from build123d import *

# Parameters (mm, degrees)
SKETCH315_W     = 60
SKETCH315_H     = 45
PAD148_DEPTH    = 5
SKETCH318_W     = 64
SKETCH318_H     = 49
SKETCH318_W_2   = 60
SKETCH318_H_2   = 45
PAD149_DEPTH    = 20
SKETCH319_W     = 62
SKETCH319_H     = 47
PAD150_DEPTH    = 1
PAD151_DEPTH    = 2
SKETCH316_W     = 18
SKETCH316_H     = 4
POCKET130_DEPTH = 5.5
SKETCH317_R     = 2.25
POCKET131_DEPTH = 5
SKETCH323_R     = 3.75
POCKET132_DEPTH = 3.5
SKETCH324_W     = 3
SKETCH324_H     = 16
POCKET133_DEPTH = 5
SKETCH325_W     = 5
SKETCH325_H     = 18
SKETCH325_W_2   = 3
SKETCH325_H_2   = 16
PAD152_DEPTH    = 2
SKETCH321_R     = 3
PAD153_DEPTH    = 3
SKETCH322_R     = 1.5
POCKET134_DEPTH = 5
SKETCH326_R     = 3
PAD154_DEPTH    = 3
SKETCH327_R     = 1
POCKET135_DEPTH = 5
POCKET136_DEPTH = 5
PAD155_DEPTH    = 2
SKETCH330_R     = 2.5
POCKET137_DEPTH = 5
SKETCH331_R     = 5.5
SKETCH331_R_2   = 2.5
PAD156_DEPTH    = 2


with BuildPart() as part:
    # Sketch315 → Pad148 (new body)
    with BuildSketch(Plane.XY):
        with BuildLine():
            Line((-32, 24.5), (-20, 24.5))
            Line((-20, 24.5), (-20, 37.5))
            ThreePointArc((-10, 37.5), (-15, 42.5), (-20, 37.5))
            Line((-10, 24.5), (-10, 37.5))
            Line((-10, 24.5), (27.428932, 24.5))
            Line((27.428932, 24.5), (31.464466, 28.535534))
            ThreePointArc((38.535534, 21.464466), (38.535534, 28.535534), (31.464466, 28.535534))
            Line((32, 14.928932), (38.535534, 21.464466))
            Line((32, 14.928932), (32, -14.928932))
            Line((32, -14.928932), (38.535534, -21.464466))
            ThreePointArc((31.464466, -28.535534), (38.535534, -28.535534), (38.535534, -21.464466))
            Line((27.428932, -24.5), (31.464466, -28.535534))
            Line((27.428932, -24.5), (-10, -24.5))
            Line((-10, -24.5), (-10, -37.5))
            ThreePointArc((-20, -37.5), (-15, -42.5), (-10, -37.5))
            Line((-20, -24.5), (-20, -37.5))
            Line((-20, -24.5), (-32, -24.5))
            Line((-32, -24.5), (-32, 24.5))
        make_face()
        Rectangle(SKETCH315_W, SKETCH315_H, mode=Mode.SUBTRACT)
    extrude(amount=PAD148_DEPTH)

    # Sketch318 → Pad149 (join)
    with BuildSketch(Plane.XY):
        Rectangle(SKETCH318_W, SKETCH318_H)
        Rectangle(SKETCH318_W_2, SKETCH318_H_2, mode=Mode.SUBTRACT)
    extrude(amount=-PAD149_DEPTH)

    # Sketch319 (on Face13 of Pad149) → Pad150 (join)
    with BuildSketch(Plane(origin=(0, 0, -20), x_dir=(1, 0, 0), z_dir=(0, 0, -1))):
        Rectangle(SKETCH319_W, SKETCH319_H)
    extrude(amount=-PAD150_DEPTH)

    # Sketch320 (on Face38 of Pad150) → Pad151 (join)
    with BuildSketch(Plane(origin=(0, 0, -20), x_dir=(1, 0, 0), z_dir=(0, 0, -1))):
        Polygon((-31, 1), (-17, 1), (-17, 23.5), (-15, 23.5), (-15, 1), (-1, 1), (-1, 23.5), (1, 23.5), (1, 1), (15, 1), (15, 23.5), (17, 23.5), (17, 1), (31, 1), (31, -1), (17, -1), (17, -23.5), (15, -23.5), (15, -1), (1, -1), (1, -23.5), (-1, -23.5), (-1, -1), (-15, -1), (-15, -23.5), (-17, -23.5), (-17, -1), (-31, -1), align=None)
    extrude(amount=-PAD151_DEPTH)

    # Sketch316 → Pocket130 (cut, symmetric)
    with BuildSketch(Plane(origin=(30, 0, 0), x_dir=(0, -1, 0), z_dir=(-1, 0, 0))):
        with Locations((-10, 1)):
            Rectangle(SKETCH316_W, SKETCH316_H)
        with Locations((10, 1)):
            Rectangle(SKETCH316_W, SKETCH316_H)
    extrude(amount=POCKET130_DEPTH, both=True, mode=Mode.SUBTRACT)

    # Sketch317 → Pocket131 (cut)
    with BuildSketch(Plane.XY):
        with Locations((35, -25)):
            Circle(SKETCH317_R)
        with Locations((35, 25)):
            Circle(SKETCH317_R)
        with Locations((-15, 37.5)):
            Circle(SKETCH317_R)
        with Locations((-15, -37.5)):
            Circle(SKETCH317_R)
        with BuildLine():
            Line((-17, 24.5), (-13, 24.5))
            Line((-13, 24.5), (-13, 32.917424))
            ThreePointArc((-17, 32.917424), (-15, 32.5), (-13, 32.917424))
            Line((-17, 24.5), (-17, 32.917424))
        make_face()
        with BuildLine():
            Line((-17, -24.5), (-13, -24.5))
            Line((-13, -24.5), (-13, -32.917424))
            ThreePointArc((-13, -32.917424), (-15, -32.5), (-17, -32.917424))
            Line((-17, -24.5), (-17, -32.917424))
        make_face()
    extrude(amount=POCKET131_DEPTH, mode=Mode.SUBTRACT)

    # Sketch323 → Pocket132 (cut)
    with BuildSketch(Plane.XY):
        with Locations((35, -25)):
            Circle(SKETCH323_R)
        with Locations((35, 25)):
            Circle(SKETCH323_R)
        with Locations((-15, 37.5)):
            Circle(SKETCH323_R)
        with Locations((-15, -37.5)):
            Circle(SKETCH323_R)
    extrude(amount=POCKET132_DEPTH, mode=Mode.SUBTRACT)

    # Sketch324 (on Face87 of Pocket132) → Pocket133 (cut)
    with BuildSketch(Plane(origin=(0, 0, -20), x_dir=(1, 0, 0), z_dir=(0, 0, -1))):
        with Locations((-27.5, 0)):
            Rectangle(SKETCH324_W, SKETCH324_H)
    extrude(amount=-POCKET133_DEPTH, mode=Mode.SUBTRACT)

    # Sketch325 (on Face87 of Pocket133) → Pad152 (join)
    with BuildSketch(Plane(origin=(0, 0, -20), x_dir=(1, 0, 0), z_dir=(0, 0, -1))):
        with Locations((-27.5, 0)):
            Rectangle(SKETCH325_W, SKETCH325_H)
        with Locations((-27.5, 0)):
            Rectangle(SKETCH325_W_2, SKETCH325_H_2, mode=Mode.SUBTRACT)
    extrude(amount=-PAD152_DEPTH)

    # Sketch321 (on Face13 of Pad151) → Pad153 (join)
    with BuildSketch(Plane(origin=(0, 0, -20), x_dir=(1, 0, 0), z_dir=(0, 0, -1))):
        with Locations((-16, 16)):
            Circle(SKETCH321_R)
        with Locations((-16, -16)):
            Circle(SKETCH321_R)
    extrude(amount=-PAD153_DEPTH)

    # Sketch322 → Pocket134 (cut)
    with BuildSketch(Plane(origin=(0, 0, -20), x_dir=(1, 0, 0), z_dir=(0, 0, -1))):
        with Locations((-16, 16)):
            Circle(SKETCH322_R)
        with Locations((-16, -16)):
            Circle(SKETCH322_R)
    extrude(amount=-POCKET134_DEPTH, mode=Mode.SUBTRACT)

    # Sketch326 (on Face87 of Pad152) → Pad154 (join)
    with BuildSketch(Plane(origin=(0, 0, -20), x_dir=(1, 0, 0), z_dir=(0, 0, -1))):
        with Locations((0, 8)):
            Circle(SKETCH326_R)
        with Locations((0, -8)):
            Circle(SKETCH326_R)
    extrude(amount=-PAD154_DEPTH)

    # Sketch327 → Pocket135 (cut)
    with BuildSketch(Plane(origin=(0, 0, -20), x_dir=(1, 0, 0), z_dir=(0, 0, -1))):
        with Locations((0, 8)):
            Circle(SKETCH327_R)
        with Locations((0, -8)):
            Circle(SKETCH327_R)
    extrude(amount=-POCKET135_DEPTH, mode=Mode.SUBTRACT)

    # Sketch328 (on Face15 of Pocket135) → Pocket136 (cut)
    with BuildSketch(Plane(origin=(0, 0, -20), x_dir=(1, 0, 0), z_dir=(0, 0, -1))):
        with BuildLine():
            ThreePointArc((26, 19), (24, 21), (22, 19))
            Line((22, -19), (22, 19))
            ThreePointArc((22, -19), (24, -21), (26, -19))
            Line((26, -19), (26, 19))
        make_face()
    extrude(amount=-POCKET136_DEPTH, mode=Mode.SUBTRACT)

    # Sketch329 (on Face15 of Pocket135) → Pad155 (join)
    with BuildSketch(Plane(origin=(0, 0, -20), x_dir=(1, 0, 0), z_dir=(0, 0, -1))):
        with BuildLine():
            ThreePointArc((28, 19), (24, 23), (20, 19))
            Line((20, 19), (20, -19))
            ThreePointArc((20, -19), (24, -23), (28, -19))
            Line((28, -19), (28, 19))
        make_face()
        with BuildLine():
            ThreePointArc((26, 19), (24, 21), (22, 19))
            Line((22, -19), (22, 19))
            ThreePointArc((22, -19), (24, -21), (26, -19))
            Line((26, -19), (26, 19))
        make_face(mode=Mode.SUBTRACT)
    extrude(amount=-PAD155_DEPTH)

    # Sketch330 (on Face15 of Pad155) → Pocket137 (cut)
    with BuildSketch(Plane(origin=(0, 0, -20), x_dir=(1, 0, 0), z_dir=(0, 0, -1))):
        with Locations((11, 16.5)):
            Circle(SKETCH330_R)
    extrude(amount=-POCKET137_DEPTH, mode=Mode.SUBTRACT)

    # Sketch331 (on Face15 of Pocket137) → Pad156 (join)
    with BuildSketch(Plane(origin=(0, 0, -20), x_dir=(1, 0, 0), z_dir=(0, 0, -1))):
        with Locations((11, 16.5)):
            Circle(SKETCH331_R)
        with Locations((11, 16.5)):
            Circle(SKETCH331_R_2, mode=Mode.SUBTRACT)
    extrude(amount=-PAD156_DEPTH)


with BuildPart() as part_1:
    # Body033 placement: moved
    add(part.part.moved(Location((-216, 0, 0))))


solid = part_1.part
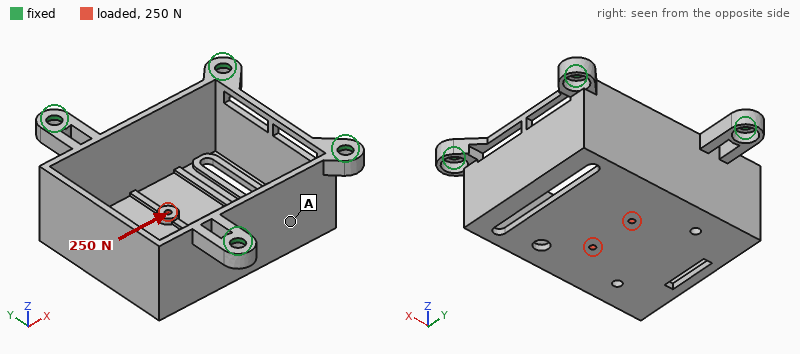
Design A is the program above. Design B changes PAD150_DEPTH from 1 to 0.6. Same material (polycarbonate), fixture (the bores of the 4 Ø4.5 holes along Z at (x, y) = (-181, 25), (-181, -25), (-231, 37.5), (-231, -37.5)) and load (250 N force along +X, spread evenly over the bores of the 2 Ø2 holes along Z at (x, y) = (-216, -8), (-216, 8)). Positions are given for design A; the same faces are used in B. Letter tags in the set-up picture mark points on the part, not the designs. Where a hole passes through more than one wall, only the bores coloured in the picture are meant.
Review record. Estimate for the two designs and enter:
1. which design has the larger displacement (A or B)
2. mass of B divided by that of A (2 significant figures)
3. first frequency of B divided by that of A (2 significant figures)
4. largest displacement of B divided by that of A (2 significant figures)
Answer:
B
0.95
1.0
1.5
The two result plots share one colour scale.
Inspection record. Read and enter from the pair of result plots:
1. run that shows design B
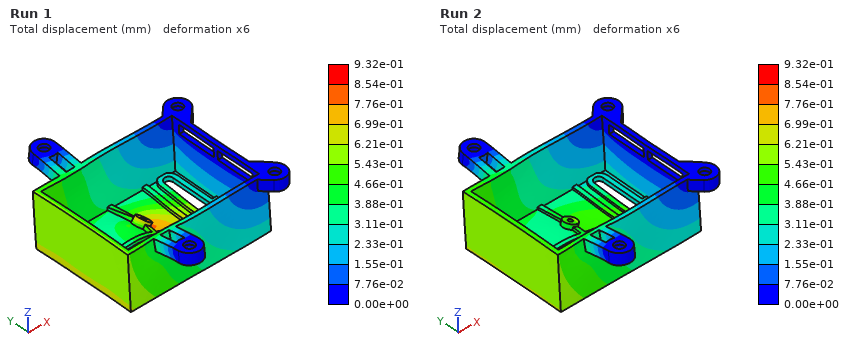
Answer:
Run 1
